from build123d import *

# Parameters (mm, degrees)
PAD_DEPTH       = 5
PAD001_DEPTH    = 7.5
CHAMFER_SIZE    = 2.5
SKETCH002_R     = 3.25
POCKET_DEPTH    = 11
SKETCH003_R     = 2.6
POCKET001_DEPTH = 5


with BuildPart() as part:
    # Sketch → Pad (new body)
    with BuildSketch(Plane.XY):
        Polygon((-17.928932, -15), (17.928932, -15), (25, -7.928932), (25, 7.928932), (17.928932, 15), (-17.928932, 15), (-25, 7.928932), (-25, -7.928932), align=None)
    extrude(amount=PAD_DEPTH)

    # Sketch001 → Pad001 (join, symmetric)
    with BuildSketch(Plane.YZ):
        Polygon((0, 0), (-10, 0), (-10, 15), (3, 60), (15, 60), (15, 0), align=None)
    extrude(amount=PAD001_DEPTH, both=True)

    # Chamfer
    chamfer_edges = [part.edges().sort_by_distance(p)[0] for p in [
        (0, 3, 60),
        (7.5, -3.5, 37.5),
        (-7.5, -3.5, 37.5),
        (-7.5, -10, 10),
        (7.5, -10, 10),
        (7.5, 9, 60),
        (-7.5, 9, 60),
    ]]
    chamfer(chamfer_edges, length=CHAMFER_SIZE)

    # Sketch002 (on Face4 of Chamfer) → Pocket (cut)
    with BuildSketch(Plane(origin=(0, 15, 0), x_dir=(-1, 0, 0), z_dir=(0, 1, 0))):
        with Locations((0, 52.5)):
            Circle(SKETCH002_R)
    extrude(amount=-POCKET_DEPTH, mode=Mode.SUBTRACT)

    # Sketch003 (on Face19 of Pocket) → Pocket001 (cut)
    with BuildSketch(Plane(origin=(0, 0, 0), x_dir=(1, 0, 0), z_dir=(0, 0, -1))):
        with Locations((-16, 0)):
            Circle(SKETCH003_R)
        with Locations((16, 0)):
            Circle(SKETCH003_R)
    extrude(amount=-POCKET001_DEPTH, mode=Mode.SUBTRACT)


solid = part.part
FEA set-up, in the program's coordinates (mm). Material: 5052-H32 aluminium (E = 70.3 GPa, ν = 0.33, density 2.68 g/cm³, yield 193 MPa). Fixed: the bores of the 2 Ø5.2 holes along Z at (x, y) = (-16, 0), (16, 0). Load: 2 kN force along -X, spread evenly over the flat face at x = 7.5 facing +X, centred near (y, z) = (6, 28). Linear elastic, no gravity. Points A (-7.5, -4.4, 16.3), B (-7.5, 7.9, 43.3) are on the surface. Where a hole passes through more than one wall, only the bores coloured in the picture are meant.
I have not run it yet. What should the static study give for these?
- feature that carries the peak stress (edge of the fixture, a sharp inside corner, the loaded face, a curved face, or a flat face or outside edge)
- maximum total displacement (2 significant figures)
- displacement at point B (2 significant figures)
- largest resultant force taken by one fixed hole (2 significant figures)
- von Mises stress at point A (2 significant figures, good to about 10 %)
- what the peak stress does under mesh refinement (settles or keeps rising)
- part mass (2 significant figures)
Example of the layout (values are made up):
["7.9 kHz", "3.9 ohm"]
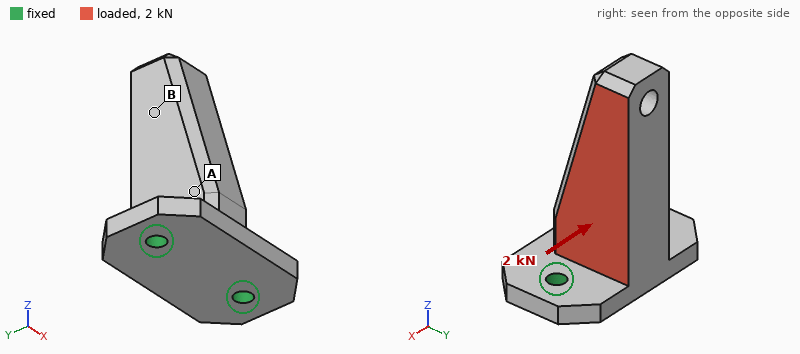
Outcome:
["edge of the fixture", "0.19 mm", "0.13 mm", "2.3 kN", "33 MPa", "keeps rising", "60 g"]
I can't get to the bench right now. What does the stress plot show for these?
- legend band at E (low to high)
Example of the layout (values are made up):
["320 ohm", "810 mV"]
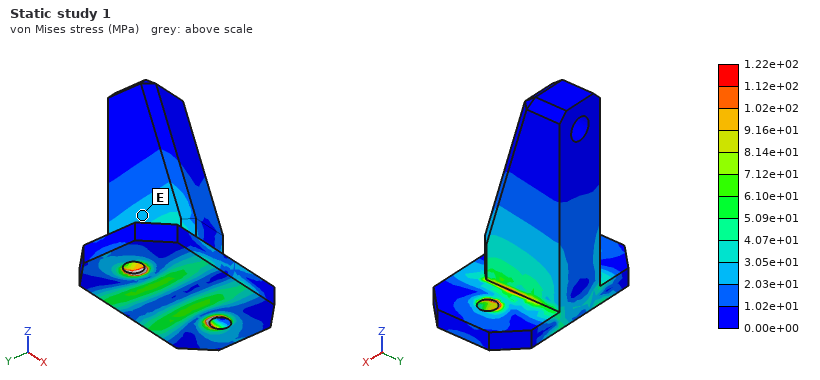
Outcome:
["2.03e+01 to 3.05e+01 MPa"]
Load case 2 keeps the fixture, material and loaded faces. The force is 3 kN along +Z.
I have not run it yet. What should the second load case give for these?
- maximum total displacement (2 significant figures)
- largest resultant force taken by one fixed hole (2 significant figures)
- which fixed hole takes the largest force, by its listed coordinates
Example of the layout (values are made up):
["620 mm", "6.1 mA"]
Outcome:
["0.18 mm", "2.5 kN", "(16, 0)"]
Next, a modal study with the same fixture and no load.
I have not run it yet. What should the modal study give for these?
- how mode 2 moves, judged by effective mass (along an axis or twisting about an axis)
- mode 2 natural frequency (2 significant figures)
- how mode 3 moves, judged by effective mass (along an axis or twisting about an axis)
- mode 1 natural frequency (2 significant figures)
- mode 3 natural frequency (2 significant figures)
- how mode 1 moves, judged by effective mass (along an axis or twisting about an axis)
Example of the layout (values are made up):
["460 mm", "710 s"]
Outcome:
["along X", "3300 Hz", "along Z", "2100 Hz", "9500 Hz", "along Y"]
